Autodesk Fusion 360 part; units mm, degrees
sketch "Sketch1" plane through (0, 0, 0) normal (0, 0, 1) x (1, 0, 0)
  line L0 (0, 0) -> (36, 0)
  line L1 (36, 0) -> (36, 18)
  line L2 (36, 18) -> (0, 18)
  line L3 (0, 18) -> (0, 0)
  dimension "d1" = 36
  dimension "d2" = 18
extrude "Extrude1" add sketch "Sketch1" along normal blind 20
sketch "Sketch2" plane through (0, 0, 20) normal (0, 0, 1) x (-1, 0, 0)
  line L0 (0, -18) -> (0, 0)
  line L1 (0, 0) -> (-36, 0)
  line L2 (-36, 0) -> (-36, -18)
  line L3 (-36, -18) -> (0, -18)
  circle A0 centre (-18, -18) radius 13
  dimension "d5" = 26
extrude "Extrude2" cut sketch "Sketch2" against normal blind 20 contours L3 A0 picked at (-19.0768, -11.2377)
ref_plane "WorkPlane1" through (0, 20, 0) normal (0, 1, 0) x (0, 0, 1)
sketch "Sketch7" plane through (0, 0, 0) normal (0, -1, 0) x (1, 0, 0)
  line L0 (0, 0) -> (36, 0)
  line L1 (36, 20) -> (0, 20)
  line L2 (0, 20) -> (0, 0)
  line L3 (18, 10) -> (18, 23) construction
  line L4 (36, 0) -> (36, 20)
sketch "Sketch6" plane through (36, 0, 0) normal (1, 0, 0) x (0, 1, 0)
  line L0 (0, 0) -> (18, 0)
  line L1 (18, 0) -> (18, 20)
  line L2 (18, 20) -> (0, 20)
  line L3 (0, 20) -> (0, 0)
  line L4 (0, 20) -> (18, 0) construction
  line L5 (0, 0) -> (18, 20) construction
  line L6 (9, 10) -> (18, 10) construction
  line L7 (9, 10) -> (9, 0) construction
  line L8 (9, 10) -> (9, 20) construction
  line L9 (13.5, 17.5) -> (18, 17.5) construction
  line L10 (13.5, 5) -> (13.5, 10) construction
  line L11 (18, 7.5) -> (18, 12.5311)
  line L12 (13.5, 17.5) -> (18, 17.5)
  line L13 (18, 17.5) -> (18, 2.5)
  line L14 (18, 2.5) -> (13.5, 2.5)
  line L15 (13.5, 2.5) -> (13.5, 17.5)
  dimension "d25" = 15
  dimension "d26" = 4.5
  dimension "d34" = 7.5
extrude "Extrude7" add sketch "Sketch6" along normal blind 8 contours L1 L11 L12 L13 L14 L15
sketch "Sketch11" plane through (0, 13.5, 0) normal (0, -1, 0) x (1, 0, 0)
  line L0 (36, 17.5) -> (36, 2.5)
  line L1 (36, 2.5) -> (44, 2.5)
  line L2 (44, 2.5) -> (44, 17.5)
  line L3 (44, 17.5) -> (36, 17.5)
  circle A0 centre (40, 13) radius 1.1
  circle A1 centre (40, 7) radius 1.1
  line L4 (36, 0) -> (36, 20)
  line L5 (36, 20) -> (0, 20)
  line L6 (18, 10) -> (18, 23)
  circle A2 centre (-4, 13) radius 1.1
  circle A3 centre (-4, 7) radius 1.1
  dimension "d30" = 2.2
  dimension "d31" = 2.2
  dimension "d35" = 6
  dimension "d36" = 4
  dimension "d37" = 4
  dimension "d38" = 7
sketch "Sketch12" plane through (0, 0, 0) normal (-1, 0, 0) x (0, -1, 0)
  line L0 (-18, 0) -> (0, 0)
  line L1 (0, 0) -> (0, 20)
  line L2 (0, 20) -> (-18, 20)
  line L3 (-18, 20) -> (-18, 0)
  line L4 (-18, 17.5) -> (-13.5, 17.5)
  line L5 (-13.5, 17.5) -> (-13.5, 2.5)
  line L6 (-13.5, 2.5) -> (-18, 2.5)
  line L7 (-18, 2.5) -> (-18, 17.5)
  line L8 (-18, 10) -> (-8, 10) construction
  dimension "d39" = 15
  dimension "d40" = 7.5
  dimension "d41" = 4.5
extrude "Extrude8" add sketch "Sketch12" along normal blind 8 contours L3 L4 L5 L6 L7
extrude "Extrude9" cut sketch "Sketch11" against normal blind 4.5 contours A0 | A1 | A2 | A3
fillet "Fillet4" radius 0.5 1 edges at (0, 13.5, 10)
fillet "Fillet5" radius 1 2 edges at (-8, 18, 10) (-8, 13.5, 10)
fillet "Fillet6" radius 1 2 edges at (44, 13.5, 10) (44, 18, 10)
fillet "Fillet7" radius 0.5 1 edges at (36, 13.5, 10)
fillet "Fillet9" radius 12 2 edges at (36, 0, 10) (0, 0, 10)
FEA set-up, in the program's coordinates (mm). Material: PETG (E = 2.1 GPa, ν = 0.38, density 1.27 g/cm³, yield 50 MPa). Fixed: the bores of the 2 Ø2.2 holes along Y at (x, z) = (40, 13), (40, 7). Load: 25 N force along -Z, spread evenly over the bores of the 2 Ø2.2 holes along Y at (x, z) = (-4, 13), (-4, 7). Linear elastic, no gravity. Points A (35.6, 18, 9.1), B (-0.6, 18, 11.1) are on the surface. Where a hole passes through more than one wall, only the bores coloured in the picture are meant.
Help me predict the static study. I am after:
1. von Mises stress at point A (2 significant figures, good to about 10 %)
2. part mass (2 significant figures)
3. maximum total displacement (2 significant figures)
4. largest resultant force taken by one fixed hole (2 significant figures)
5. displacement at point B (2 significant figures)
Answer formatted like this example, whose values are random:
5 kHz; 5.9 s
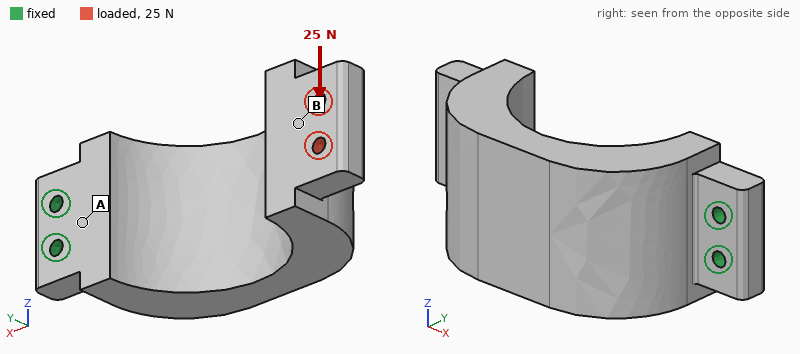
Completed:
6.6 MPa; 9.4 g; 0.70 mm; 140 N; 0.59 mm
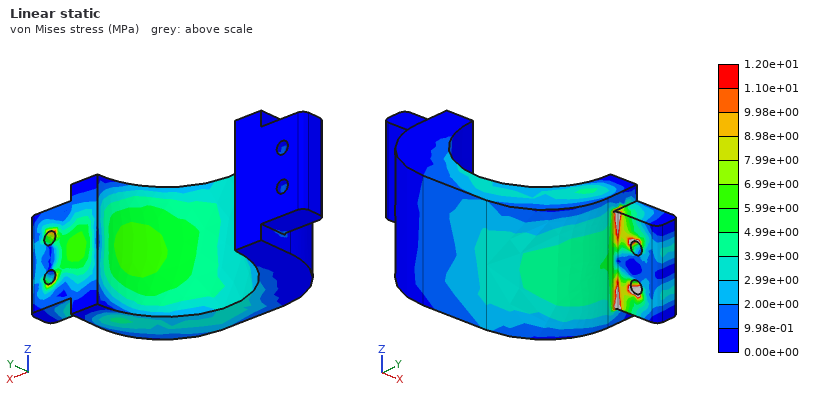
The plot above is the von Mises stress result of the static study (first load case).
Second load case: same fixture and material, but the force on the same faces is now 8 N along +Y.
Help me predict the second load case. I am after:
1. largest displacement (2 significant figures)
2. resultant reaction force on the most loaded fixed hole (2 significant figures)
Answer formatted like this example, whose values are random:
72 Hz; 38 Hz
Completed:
0.63 mm; 5.2 N
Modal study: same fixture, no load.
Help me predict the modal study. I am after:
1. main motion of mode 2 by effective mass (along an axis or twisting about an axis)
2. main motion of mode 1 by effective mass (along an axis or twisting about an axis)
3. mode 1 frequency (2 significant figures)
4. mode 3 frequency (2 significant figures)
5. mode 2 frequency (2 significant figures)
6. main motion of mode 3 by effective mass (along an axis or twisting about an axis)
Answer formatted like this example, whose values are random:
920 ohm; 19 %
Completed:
along Z; along Y; 360 Hz; 1300 Hz; 660 Hz; along X
